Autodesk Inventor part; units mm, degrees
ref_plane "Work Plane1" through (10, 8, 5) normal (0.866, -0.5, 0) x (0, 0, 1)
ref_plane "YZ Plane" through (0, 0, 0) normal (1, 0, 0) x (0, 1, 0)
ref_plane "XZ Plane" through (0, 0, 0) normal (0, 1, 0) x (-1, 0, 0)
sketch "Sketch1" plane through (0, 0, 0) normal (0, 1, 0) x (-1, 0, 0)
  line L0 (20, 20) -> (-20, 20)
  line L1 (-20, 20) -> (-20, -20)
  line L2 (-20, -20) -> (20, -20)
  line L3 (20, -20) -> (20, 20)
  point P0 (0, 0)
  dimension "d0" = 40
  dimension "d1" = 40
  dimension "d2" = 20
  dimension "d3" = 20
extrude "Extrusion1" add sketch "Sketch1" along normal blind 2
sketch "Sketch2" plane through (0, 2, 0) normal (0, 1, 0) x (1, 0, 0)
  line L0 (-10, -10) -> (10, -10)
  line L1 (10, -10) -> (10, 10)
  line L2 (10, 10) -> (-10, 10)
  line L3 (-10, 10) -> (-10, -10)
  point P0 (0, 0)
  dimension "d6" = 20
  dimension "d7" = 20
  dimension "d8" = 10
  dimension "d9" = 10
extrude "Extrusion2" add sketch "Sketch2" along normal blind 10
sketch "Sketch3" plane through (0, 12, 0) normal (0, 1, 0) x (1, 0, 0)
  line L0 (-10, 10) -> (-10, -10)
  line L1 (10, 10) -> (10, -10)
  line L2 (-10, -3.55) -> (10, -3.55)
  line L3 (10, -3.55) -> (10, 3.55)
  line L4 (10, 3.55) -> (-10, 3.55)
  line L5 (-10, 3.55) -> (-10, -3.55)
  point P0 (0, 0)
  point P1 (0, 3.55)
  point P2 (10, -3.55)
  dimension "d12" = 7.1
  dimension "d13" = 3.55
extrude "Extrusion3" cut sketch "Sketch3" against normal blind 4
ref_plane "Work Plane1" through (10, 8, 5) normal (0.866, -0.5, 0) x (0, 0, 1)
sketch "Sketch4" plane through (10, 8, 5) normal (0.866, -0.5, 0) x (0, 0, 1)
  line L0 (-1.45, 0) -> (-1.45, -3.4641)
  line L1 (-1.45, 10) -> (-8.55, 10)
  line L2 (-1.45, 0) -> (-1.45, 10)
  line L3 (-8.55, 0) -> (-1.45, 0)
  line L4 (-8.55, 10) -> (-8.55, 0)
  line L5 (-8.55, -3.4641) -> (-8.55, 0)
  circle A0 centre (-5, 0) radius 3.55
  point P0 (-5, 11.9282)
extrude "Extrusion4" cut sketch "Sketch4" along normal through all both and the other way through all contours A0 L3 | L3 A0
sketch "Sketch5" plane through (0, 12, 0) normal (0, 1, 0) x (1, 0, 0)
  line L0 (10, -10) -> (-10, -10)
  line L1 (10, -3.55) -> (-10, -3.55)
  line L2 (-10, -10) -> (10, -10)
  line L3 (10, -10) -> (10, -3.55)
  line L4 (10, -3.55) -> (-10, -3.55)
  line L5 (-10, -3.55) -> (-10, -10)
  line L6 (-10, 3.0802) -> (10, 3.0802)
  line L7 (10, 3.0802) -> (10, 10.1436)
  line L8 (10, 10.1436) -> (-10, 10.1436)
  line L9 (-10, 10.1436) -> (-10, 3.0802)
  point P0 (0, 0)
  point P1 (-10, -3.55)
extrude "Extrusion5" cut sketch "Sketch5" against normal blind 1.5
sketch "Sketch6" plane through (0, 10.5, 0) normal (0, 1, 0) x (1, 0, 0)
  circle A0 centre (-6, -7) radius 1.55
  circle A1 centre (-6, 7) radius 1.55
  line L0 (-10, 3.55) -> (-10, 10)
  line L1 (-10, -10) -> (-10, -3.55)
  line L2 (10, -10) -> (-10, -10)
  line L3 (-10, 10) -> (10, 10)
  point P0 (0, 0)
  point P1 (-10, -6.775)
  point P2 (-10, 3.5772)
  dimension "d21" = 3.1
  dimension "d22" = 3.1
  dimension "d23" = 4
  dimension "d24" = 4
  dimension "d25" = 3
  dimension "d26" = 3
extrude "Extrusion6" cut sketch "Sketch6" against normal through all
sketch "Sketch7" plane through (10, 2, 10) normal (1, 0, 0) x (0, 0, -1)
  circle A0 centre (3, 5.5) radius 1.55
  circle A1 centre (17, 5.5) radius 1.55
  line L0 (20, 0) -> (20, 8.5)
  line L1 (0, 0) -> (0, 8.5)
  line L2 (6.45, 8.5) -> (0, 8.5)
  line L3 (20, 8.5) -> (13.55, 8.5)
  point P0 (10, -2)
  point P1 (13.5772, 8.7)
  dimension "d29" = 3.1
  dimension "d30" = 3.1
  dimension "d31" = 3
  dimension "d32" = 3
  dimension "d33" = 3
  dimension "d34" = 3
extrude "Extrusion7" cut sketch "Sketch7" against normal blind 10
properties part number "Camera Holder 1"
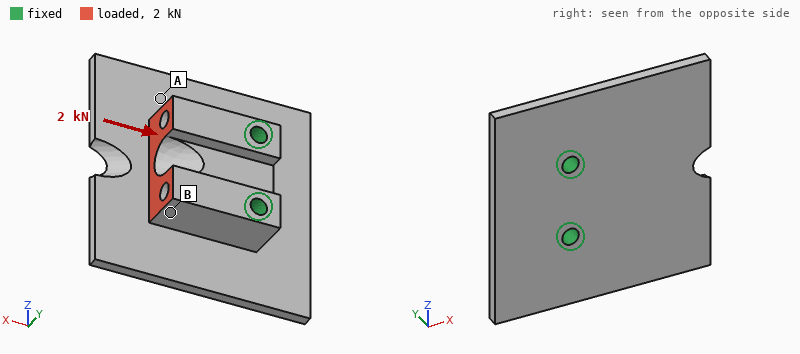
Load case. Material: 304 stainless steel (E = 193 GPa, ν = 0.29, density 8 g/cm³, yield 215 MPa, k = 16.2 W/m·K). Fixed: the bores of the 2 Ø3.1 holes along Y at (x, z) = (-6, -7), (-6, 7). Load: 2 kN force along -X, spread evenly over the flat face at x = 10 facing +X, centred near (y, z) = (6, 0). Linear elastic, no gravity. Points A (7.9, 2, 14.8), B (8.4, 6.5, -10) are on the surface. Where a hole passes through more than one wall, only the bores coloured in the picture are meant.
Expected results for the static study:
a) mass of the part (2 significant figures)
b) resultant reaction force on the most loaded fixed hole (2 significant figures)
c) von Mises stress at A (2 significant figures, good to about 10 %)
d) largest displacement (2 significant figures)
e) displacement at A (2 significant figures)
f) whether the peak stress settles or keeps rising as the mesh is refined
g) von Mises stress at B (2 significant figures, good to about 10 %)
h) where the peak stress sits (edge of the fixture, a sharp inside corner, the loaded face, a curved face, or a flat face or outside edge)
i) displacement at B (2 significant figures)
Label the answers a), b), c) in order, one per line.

a) 47 g
b) 1.0 kN
c) 3.1 MPa
d) 2.4 µm
e) 0.56 µm
f) keeps rising
g) 18 MPa
h) edge of the fixture
i) 1.3 µm
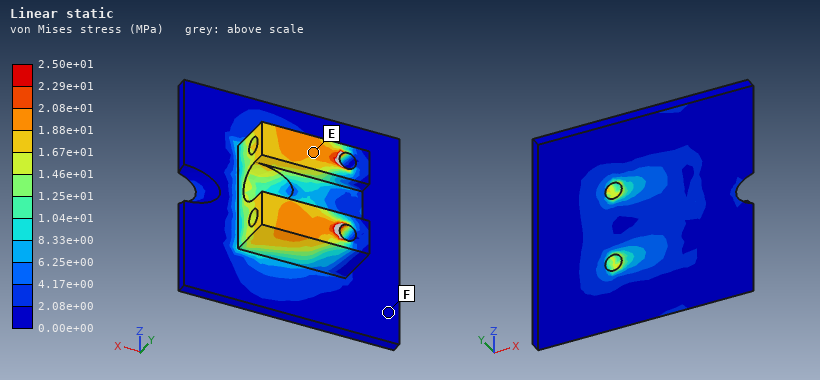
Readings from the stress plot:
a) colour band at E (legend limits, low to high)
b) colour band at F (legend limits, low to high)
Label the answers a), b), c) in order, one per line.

a) 1.88e+01 to 2.08e+01 MPa
b) 0.00e+00 to 2.08e+00 MPa
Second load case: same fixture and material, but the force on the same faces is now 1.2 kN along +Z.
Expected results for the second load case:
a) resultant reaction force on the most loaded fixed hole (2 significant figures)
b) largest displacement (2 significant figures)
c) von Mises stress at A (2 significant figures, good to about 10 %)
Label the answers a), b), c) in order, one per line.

a) 1.3 kN
b) 4.9 µm
c) 5.5 MPa
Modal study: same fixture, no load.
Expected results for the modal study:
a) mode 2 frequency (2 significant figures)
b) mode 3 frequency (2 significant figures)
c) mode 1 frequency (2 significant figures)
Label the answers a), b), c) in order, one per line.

a) 8300 Hz
b) 9300 Hz
c) 8300 Hz
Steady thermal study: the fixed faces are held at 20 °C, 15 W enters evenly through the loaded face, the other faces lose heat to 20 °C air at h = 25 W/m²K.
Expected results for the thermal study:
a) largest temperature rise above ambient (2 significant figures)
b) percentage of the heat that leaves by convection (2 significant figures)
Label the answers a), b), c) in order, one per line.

a) 81 K
b) 17 %
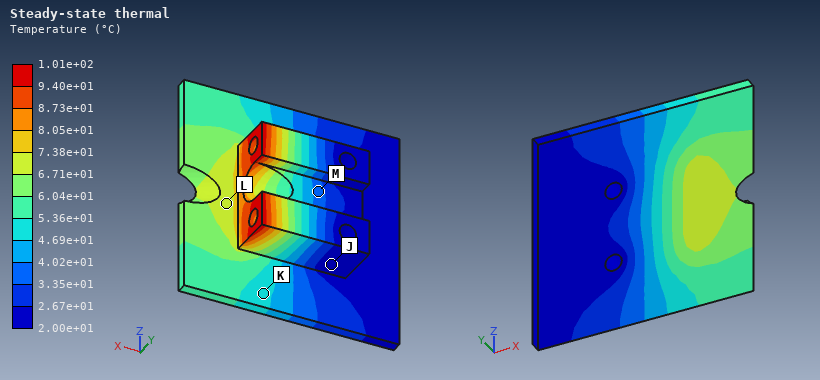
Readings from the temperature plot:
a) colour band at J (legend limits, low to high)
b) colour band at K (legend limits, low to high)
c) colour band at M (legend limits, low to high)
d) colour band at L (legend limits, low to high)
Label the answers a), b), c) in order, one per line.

a) 2.00e+01 to 2.67e+01 °C
b) 4.69e+01 to 5.36e+01 °C
c) 3.35e+01 to 4.02e+01 °C
d) 6.71e+01 to 7.38e+01 °C
